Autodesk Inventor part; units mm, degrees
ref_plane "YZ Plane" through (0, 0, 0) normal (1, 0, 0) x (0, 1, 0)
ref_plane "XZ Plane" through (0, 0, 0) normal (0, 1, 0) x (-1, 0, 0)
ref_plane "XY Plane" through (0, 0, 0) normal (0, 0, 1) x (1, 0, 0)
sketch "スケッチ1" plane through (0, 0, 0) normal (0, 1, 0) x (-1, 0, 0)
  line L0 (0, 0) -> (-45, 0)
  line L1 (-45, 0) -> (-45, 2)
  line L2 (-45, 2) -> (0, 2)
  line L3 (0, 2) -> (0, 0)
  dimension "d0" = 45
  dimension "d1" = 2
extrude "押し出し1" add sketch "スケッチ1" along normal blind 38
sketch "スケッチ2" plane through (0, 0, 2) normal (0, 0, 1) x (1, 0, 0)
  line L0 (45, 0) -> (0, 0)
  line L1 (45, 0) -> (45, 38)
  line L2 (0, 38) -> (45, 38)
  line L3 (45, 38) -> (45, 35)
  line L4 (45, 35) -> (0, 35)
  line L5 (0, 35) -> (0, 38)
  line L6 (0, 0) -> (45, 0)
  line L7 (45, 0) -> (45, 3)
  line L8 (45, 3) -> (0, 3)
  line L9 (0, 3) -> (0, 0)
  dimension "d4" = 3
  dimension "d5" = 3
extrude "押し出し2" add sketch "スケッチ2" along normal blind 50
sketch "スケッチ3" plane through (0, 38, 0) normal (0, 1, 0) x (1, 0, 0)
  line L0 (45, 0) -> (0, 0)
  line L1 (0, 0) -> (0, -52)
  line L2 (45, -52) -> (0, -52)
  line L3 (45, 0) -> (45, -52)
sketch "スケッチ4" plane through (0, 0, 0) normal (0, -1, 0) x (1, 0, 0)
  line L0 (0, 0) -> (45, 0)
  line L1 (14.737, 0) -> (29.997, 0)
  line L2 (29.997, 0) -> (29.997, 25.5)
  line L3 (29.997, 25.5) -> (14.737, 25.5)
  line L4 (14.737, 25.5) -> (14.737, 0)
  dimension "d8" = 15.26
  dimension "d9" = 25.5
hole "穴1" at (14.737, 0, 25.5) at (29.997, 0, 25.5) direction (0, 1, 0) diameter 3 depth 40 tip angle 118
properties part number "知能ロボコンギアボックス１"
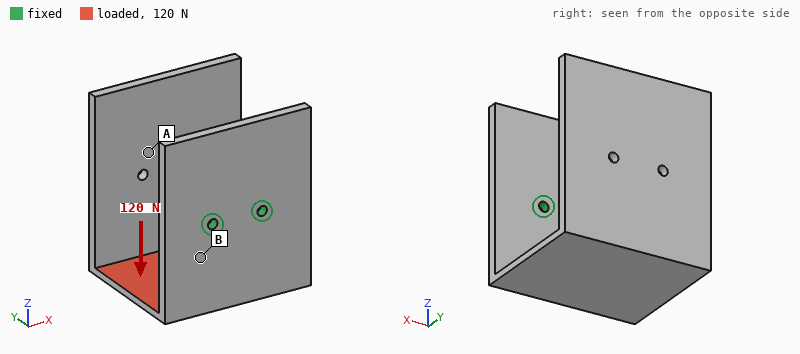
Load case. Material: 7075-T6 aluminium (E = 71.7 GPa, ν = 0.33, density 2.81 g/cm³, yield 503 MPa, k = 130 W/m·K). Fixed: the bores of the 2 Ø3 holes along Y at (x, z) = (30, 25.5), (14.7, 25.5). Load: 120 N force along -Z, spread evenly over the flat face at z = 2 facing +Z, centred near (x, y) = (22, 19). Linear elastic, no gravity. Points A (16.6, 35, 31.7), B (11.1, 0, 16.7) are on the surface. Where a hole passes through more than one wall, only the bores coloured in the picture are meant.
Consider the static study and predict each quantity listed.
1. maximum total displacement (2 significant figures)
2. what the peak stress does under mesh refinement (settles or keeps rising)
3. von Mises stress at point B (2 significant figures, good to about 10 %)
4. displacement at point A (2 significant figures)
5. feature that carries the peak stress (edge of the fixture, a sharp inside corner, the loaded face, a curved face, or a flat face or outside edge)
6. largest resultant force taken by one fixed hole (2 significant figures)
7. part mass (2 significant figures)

0.89 mm
keeps rising
27 MPa
0.61 mm
edge of the fixture
62 N
47 g
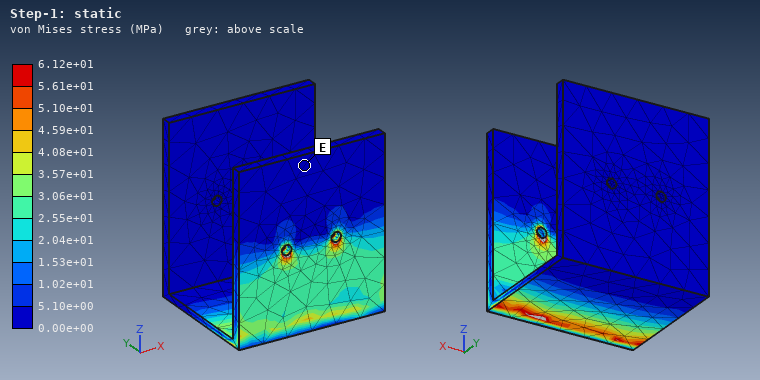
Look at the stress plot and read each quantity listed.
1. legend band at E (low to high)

0.00e+00 to 5.10e+00 MPa
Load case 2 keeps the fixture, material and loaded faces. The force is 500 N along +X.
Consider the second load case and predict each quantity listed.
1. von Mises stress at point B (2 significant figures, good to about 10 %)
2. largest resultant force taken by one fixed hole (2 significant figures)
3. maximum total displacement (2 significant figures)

68 MPa
830 N
0.93 mm
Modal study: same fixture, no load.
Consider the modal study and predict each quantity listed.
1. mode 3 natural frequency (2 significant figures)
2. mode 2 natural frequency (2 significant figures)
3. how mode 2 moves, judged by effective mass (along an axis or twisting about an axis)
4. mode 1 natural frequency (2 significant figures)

660 Hz
390 Hz
along X
240 Hz
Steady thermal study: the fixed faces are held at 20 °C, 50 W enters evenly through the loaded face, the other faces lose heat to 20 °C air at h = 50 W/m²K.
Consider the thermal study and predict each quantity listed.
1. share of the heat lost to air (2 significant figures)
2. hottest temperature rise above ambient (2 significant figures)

47 %
74 K
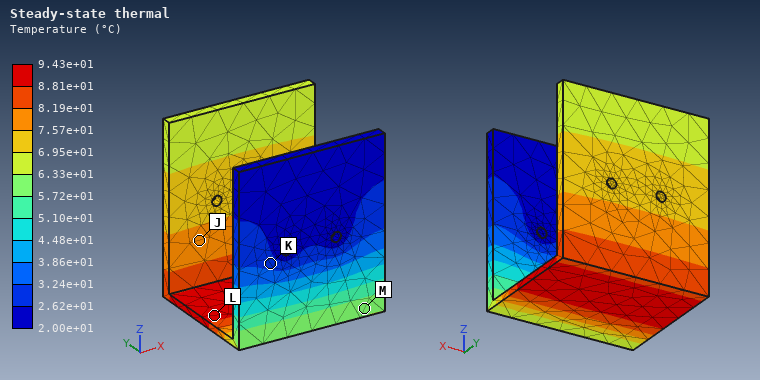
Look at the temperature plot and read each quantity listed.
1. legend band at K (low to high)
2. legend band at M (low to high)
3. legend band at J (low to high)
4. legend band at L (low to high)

2.62e+01 to 3.24e+01 °C
5.72e+01 to 6.33e+01 °C
7.57e+01 to 8.19e+01 °C
8.81e+01 to 9.43e+01 °C
